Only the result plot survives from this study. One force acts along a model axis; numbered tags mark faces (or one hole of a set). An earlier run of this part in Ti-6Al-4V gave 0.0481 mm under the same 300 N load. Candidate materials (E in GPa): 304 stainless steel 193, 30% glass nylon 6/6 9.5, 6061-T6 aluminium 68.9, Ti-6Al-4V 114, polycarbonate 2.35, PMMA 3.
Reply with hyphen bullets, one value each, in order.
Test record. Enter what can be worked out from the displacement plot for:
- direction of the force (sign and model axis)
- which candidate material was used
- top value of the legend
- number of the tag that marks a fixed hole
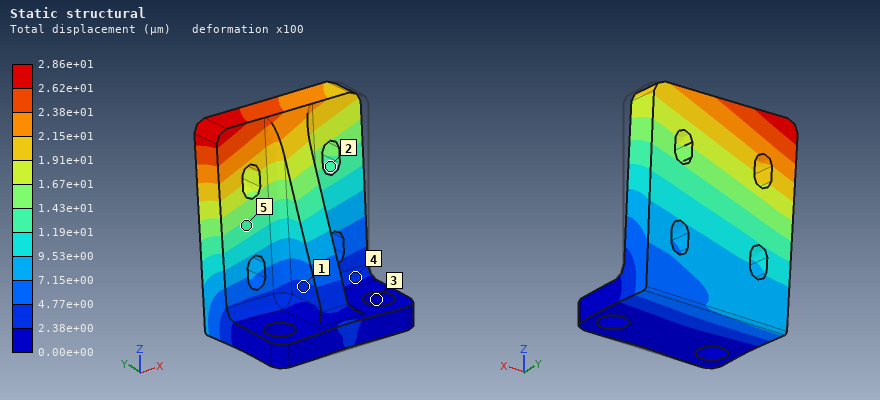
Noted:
- +Y
- 304 stainless steel
- 2.86e+01 µm
- 3
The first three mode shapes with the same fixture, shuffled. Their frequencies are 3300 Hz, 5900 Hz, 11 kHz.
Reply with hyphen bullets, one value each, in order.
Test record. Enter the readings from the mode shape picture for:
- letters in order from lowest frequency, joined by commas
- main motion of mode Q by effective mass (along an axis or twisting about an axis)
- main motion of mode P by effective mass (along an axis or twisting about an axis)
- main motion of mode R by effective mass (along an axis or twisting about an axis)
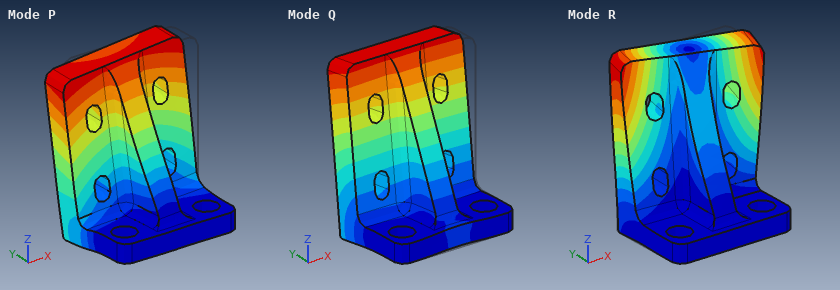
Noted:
- Q, P, R
- along Y
- along X
- twisting about Z
